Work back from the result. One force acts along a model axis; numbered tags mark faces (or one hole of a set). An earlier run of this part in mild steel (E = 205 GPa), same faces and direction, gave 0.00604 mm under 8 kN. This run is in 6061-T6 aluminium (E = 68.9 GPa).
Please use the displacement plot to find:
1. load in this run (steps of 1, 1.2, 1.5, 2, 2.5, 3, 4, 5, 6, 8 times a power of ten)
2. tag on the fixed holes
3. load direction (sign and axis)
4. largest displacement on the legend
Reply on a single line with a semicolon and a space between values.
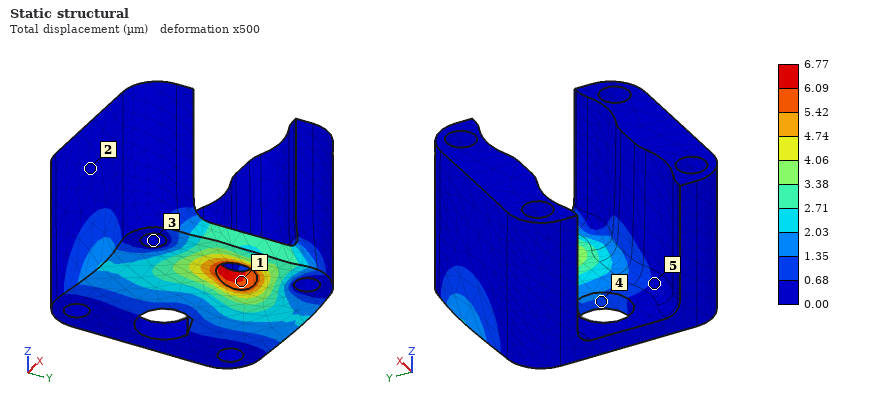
3 kN; 3; +Y; 6.77 µm
